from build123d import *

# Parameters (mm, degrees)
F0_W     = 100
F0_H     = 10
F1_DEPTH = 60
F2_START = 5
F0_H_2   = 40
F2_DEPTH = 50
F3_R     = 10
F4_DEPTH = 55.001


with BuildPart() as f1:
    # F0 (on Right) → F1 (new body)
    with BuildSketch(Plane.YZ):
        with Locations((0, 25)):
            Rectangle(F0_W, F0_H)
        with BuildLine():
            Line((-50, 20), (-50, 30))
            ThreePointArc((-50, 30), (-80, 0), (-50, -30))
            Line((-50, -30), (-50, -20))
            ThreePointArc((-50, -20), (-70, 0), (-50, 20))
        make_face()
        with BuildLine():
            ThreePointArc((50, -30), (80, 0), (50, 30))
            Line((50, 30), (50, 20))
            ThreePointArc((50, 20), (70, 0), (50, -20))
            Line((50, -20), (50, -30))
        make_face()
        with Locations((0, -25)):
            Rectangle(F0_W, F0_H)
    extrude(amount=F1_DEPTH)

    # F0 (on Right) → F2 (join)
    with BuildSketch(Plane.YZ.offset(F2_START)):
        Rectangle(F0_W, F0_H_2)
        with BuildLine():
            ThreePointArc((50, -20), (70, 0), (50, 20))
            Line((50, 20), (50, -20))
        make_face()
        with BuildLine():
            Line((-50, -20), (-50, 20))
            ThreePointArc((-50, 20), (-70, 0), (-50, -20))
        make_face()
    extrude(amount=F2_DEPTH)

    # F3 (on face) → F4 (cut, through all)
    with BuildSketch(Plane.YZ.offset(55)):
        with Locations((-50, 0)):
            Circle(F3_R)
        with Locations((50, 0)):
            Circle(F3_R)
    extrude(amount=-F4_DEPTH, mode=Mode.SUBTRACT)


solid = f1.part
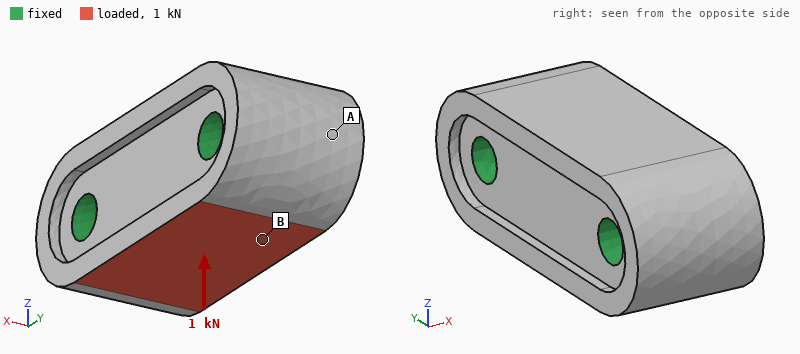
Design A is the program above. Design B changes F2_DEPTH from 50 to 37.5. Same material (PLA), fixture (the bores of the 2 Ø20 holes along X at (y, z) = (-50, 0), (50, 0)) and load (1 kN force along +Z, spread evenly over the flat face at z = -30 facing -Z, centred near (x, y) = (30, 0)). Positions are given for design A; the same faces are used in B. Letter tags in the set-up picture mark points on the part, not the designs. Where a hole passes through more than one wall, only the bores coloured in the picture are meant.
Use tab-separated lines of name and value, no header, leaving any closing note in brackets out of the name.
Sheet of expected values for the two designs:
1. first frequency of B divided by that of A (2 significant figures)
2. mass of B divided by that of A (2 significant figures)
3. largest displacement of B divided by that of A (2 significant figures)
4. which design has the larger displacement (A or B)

first frequency of B divided by that of A	0.80
mass of B divided by that of A	0.87
largest displacement of B divided by that of A	4.5
which design has the larger displacement	B
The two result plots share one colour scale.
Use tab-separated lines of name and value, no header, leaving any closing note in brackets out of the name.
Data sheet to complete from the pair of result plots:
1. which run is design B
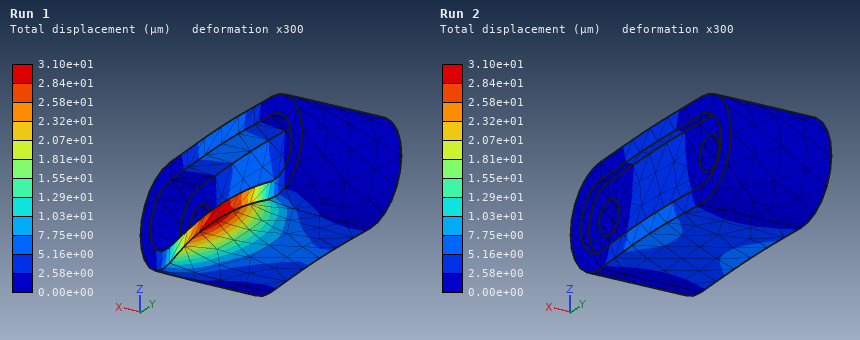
which run is design B	Run 1
